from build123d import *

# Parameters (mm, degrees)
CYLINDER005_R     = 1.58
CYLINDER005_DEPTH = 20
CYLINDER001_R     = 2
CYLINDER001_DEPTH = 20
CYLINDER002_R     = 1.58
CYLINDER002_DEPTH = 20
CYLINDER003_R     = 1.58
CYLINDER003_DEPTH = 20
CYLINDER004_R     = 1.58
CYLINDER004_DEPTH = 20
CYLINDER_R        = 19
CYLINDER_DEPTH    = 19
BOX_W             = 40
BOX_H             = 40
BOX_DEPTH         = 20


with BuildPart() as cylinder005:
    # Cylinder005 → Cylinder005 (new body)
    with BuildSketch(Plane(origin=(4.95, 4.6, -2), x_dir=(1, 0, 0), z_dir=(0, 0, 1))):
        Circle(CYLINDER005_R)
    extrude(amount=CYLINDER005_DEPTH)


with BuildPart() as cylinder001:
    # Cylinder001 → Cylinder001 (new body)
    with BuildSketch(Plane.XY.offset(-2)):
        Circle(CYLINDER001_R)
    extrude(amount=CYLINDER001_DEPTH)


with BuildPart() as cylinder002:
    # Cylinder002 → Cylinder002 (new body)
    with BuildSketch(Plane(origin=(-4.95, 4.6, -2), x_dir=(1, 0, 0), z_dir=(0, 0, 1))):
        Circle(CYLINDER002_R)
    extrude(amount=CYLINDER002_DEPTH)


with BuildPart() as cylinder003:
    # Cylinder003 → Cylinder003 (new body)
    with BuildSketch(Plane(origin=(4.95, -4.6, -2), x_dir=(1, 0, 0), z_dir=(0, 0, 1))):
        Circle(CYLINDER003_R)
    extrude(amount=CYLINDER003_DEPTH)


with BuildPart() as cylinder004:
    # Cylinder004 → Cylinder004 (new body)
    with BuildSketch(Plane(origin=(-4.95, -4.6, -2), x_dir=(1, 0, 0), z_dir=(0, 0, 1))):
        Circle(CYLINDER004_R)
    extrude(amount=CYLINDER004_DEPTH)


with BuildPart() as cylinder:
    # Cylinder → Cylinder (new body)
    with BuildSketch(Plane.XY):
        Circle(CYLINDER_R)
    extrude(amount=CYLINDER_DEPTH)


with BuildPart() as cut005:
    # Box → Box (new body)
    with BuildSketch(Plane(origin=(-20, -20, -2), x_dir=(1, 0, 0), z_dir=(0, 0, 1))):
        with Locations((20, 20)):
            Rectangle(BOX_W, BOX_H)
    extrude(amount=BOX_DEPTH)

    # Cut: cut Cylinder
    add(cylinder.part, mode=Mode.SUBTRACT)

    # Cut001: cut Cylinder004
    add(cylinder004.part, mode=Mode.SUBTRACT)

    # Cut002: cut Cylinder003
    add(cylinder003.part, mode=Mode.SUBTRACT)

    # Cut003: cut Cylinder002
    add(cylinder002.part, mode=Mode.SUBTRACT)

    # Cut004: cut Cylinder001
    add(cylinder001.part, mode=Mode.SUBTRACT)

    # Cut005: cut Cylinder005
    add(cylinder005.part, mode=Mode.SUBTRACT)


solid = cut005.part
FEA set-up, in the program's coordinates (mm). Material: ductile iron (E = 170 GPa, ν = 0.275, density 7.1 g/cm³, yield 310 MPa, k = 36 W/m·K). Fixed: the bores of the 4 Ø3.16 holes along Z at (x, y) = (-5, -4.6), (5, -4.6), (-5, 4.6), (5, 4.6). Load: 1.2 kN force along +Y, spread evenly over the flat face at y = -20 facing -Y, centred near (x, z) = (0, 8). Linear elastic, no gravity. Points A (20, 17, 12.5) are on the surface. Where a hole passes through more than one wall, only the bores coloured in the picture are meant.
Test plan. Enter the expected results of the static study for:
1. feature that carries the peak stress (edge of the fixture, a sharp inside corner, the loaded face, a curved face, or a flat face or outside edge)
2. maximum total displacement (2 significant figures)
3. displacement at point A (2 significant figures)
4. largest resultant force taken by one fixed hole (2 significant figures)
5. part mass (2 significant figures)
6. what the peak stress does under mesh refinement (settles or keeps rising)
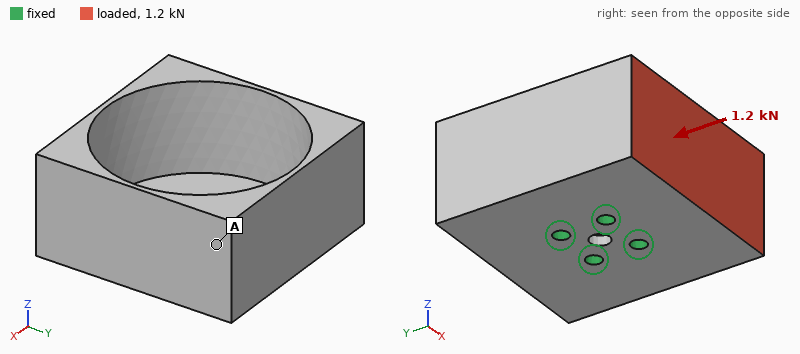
edge of the fixture
83 µm
53 µm
540 N
82 g
keeps rising
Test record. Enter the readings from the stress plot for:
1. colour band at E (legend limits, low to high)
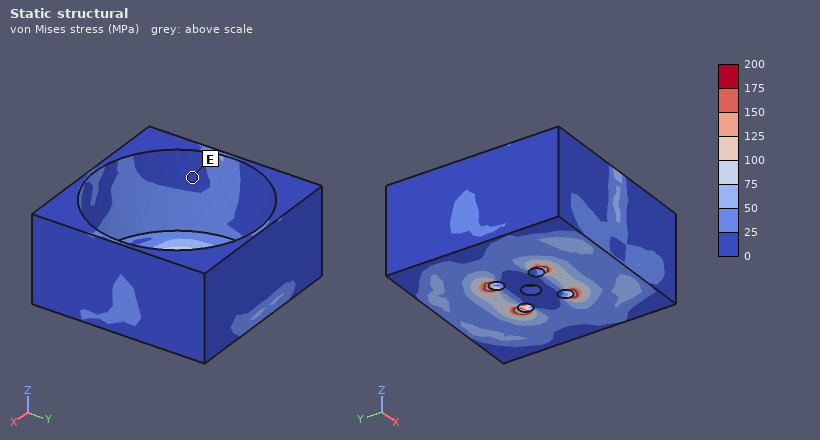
0 to 25 MPa
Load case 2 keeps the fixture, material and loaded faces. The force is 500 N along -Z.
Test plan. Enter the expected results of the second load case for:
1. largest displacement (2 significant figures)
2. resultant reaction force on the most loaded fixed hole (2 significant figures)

68 µm
420 N
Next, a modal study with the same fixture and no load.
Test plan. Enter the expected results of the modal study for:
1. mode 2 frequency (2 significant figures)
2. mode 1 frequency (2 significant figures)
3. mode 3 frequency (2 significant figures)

2300 Hz
2200 Hz
3200 Hz
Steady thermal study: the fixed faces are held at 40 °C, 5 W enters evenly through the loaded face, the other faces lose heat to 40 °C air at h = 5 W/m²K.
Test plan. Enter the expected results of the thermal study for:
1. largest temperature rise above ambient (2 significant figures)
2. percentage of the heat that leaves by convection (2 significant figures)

26 K
7.8 %
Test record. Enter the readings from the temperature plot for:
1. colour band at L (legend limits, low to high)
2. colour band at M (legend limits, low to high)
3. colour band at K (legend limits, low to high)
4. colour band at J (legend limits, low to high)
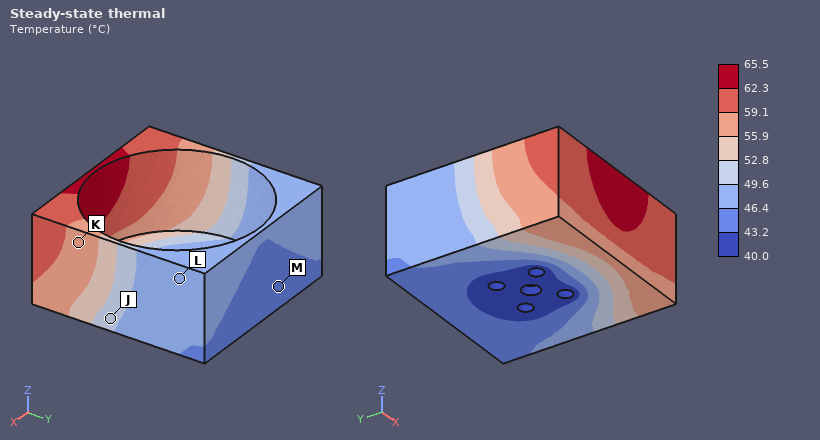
46.4 to 49.6 °C
43.2 to 46.4 °C
55.9 to 59.1 °C
49.6 to 52.8 °C
